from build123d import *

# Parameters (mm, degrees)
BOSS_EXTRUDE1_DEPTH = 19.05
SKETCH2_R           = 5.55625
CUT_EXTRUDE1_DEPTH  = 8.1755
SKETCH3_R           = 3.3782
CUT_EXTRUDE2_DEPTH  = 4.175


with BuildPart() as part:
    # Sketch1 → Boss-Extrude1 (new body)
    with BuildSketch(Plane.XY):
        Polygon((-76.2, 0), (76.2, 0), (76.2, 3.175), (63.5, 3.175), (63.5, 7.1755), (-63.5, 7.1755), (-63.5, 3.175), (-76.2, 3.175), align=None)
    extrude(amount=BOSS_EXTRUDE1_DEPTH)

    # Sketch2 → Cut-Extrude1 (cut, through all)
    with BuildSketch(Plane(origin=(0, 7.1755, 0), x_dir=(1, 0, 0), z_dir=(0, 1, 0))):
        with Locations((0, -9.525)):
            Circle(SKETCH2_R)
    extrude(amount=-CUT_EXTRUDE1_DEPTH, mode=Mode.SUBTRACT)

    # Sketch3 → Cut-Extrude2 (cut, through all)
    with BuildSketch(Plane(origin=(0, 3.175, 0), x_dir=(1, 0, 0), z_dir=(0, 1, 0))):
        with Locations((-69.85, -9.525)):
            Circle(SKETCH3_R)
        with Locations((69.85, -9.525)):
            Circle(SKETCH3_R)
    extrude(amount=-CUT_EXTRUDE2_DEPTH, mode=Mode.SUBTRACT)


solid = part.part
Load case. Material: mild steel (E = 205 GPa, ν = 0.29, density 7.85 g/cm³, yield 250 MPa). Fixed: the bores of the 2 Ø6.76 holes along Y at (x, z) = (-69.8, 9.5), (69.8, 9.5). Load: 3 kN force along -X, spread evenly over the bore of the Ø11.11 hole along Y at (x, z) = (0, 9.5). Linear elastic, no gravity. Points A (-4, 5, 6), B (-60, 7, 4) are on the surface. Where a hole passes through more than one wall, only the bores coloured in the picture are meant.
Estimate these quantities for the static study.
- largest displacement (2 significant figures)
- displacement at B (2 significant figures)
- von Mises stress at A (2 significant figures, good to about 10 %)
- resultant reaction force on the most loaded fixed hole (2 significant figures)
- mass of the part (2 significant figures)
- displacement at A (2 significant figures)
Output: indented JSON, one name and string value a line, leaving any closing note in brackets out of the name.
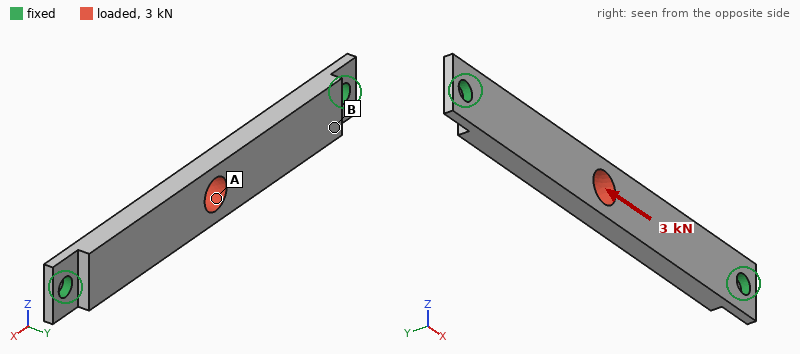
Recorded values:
{
  "largest displacement": "6.1 µm",
  "displacement at B": "3.6 µm",
  "von Mises stress at A": "17 MPa",
  "resultant reaction force on the most loaded fixed hole": "1.5 kN",
  "mass of the part": "140 g",
  "displacement at A": "4.8 µm"
}
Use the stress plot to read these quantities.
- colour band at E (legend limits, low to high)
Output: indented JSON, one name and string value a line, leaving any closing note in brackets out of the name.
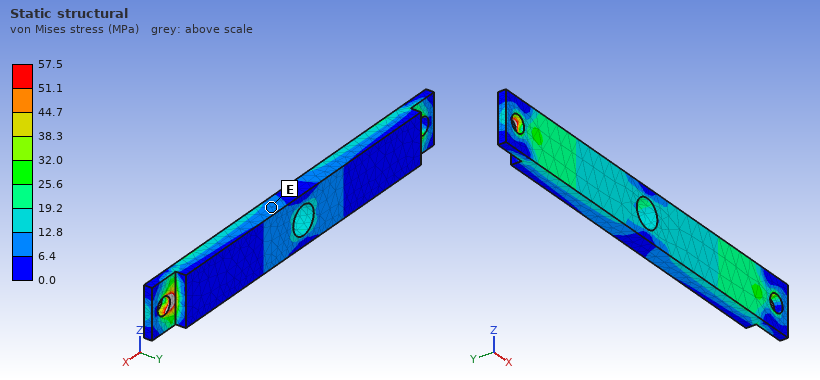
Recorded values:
{
  "colour band at E": "6.4 to 12.8 MPa"
}
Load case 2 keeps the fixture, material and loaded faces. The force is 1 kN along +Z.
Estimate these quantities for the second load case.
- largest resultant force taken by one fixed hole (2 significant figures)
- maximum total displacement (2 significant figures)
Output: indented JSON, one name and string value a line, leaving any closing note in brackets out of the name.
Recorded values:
{
  "largest resultant force taken by one fixed hole": "500 N",
  "maximum total displacement": "34 µm"
}
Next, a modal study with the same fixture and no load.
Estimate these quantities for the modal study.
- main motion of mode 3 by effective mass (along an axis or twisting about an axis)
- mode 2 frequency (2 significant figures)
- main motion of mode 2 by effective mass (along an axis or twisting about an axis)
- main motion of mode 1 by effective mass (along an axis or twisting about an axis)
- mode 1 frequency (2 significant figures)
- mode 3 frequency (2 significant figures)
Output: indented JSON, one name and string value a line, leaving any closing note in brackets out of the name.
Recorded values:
{
  "main motion of mode 3 by effective mass": "twisting about Z",
  "mode 2 frequency": "3500 Hz",
  "main motion of mode 2 by effective mass": "along Z",
  "main motion of mode 1 by effective mass": "along Y",
  "mode 1 frequency": "1400 Hz",
  "mode 3 frequency": "4100 Hz"
}
